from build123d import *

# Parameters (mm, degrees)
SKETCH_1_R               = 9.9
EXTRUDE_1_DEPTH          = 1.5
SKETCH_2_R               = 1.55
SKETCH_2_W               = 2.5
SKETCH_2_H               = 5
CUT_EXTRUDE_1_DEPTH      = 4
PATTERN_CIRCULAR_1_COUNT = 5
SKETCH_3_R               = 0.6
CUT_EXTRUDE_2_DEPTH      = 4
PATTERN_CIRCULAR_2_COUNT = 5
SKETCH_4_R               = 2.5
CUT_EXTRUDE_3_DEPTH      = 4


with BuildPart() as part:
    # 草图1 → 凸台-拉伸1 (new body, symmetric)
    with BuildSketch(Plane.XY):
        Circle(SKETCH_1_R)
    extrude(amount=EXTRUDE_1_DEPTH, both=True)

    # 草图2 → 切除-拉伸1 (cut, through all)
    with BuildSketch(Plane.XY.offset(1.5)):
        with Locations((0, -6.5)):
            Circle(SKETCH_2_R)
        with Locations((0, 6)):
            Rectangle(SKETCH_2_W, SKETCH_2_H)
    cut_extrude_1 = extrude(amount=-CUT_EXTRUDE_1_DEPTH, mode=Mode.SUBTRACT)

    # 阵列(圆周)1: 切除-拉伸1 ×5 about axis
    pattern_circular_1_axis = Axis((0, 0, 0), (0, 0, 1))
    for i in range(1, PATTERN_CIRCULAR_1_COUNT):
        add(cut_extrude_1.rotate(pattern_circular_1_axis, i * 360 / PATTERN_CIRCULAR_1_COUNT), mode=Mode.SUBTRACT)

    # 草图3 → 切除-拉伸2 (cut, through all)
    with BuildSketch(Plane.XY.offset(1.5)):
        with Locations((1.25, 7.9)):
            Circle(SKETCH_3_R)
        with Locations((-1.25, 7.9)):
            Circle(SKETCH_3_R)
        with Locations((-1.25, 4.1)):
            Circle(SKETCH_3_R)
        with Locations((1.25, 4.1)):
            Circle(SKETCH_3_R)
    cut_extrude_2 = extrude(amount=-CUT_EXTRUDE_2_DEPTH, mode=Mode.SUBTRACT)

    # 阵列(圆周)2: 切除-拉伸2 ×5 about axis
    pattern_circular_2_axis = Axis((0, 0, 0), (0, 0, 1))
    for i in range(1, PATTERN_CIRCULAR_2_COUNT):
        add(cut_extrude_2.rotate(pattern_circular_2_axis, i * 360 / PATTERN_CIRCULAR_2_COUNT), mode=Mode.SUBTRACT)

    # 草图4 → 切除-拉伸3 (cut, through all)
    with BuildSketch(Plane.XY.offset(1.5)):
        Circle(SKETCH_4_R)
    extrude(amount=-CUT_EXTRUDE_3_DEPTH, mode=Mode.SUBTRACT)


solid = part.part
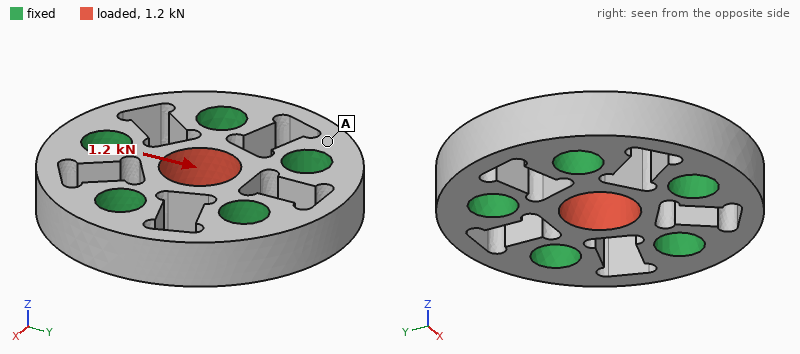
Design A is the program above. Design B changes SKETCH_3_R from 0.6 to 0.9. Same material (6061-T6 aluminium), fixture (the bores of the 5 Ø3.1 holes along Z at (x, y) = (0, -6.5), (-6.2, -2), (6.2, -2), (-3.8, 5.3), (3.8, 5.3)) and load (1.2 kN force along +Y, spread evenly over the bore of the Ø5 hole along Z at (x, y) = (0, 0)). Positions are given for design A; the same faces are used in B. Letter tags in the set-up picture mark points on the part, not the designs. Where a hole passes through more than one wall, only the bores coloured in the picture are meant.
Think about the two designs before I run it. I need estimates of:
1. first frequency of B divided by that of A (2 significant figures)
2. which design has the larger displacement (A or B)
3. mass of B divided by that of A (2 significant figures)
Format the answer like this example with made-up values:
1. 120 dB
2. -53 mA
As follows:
1. 0.97
2. B
3. 0.90
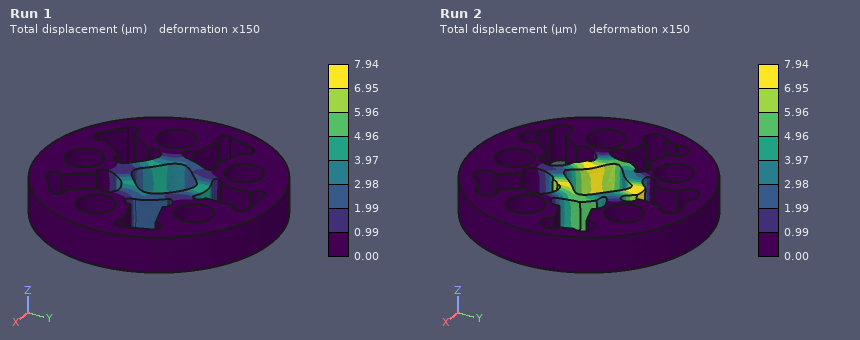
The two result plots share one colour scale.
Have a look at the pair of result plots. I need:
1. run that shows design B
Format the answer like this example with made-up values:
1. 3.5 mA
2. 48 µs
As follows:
1. Run 2
